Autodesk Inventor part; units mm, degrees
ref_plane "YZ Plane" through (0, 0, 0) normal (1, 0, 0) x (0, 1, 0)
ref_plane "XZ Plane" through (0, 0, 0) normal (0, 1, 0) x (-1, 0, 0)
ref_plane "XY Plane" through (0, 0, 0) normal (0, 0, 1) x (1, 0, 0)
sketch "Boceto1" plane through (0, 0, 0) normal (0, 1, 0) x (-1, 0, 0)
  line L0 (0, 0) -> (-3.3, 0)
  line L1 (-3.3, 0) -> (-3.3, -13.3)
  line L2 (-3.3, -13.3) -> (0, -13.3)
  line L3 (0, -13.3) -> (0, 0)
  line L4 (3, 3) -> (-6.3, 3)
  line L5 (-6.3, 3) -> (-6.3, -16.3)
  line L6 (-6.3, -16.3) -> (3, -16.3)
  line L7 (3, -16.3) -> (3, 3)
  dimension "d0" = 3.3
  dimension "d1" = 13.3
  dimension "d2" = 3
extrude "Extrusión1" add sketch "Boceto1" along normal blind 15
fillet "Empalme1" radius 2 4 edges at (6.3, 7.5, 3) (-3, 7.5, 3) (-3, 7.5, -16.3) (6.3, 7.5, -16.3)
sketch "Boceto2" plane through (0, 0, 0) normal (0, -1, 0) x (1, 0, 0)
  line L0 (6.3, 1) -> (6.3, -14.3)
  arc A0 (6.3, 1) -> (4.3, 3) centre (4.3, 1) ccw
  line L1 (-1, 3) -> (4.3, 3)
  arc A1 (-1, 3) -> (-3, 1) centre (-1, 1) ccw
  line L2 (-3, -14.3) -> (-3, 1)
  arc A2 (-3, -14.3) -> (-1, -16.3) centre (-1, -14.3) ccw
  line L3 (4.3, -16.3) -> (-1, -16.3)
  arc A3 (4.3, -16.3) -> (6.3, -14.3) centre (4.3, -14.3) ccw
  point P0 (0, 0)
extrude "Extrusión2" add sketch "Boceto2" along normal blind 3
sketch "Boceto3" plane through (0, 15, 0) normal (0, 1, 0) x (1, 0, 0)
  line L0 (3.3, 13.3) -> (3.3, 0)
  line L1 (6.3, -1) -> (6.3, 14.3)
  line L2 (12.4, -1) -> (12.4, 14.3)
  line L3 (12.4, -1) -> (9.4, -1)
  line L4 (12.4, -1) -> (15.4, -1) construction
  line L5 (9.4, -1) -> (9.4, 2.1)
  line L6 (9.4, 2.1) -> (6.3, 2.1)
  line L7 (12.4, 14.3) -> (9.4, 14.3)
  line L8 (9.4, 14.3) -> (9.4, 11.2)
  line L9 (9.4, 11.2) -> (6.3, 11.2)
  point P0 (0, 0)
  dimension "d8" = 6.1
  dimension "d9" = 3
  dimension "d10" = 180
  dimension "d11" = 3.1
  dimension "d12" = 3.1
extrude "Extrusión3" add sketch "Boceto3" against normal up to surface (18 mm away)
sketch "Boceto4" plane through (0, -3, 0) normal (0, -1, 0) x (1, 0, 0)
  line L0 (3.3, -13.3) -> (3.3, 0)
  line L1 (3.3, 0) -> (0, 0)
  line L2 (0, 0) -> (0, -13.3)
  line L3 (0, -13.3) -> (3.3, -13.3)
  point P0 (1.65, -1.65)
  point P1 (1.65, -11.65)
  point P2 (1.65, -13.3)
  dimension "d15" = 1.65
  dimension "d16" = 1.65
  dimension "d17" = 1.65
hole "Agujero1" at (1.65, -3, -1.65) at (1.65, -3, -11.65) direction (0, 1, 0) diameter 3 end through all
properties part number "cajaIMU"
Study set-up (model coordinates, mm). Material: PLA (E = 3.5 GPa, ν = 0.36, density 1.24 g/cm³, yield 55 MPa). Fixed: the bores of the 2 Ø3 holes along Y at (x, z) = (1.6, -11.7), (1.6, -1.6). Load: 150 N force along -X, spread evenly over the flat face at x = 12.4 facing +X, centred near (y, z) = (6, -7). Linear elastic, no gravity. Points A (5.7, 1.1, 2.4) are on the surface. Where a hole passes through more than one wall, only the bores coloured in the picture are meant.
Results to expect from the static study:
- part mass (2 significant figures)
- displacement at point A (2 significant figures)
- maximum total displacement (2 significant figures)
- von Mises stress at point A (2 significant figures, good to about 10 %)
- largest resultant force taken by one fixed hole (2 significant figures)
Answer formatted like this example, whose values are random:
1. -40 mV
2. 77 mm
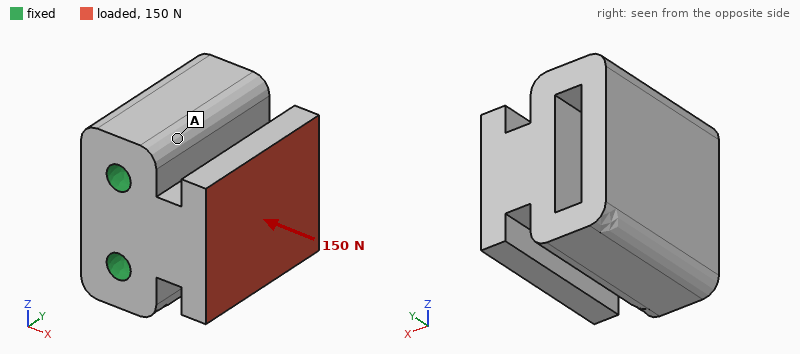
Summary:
1. 4.7 g
2. 0.031 mm
3. 0.16 mm
4. 2.7 MPa
5. 76 N
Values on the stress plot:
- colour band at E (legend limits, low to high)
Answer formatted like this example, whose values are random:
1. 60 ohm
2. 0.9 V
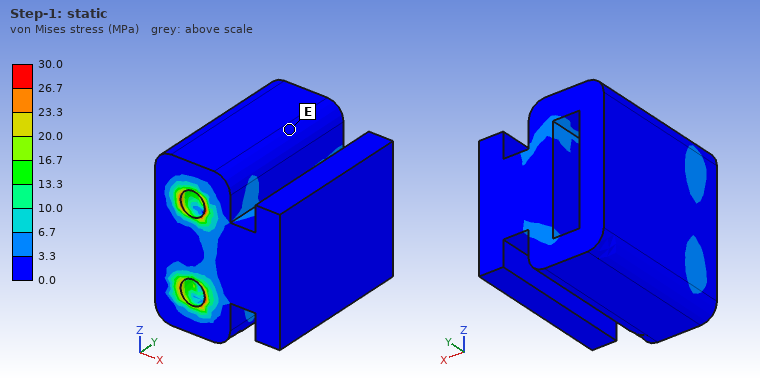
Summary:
1. 0.0 to 3.3 MPa
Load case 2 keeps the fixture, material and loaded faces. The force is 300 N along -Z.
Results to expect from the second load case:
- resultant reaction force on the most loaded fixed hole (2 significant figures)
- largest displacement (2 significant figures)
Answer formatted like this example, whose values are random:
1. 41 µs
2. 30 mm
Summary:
1. 360 N
2. 0.14 mm
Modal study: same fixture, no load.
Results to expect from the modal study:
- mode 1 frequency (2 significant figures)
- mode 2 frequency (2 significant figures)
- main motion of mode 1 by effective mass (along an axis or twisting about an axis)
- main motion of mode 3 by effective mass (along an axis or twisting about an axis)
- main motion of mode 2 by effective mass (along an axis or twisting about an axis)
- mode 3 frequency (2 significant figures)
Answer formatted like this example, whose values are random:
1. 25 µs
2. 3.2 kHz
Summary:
1. 2800 Hz
2. 6100 Hz
3. along X
4. twisting about Y
5. along Z
6. 8600 Hz
